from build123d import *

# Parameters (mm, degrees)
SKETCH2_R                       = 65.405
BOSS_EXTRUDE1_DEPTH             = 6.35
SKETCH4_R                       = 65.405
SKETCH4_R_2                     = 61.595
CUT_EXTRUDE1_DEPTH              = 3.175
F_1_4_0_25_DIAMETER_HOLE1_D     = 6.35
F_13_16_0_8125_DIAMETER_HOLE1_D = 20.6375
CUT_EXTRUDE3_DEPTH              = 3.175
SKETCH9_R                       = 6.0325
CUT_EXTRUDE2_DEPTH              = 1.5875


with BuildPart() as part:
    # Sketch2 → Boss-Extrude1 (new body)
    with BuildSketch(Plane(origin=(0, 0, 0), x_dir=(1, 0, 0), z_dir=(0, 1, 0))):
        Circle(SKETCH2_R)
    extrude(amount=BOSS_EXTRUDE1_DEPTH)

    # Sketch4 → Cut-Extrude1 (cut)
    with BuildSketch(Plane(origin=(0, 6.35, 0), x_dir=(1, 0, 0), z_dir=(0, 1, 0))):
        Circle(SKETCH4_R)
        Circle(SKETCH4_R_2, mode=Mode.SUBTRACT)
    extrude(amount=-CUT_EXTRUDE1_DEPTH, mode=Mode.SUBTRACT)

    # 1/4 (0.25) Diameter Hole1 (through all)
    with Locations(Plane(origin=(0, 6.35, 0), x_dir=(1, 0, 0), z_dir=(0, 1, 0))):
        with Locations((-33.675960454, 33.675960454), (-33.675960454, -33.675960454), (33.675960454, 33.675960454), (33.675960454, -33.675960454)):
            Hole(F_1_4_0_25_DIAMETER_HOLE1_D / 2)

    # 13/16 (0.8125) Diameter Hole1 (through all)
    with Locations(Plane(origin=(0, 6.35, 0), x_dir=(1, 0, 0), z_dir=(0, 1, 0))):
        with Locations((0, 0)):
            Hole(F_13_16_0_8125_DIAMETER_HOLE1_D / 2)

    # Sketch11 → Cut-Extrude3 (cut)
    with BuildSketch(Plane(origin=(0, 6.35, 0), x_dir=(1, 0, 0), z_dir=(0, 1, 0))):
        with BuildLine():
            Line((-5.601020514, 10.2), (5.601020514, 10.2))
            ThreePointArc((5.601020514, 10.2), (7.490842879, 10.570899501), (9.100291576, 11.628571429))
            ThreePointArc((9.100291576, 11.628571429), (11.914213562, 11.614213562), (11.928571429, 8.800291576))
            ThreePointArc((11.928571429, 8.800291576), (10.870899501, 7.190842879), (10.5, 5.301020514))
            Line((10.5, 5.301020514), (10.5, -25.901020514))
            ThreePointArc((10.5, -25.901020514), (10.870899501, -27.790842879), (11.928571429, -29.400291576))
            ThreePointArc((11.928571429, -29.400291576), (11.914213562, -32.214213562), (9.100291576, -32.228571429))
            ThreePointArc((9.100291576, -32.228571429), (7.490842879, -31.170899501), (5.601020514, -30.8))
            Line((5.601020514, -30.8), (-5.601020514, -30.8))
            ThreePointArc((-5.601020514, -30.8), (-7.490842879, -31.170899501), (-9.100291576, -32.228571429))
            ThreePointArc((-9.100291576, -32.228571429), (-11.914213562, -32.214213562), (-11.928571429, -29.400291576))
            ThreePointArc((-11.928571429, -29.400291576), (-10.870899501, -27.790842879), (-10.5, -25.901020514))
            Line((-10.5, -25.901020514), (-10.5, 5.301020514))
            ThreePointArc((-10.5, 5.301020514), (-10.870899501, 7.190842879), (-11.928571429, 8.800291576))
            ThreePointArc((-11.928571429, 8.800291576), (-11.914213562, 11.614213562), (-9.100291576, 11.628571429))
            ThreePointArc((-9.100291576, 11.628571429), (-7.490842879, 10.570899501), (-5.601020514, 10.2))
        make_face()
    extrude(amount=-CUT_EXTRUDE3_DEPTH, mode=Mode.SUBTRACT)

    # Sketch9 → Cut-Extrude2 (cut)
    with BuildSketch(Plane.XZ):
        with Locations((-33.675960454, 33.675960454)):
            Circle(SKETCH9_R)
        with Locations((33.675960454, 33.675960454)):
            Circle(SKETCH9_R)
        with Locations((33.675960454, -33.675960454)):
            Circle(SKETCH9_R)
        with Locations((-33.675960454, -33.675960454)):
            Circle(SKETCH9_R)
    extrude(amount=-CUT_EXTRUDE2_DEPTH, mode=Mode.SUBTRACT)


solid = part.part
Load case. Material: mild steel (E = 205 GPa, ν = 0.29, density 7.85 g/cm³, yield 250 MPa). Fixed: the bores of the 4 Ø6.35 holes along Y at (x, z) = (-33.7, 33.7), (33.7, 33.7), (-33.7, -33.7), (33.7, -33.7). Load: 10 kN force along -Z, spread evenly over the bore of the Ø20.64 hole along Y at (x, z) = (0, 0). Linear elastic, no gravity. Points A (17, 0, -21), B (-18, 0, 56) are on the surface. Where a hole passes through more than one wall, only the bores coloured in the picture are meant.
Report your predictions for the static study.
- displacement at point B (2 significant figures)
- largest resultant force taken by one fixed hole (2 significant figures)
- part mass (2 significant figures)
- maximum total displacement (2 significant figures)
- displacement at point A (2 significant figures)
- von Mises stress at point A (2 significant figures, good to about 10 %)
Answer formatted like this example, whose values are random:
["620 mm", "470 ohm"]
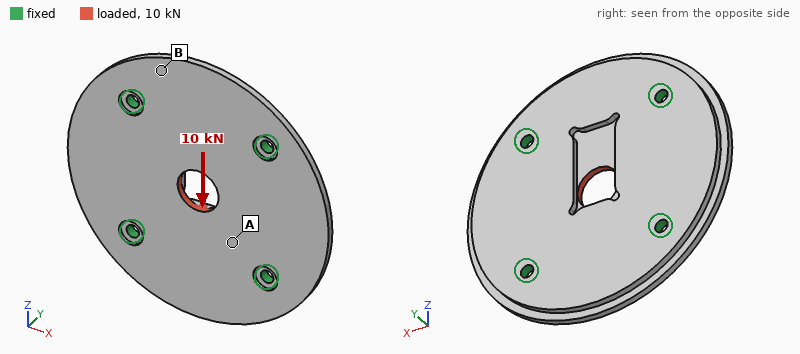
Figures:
["3.3 µm", "2.7 kN", "590 g", "6.2 µm", "2.6 µm", "20 MPa"]
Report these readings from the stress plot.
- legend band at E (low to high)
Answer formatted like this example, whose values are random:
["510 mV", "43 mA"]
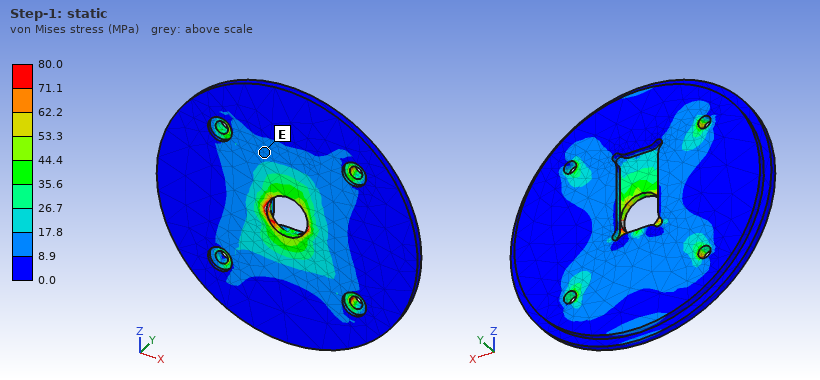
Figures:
["8.9 to 17.8 MPa"]
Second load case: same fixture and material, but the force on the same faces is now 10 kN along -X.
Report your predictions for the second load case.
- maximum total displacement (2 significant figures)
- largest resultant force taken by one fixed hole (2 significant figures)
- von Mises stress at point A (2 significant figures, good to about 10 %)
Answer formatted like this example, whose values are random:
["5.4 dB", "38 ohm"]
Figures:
["7.4 µm", "2.8 kN", "21 MPa"]
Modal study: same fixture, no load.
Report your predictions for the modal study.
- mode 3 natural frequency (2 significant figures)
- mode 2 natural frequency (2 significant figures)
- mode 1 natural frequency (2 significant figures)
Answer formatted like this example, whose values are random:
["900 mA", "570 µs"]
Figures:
["4300 Hz", "4300 Hz", "3800 Hz"]
